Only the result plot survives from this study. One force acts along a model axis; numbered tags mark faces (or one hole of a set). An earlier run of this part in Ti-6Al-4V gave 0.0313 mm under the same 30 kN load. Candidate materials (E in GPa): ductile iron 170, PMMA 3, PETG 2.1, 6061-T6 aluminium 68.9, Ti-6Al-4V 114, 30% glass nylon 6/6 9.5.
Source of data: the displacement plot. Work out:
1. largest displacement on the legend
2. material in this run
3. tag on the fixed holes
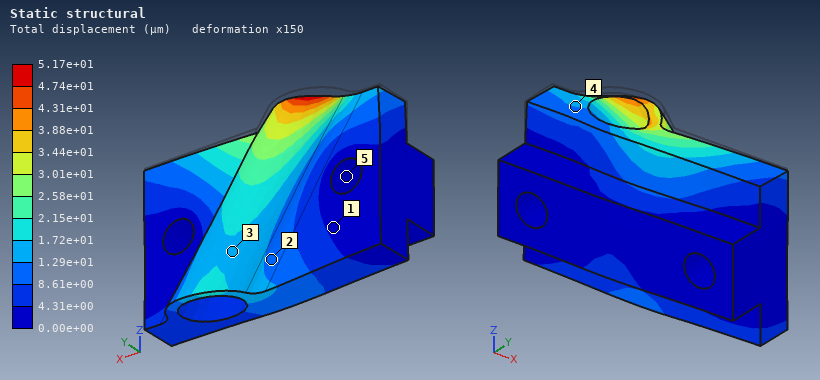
5.17e+01 µm
6061-T6 aluminium
5
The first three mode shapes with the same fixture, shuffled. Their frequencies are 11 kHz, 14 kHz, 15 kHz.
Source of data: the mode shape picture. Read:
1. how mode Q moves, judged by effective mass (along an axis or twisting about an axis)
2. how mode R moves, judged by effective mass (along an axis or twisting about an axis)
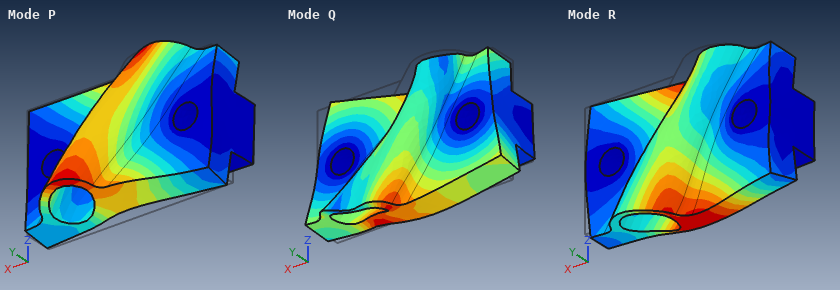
along Z
along Y
